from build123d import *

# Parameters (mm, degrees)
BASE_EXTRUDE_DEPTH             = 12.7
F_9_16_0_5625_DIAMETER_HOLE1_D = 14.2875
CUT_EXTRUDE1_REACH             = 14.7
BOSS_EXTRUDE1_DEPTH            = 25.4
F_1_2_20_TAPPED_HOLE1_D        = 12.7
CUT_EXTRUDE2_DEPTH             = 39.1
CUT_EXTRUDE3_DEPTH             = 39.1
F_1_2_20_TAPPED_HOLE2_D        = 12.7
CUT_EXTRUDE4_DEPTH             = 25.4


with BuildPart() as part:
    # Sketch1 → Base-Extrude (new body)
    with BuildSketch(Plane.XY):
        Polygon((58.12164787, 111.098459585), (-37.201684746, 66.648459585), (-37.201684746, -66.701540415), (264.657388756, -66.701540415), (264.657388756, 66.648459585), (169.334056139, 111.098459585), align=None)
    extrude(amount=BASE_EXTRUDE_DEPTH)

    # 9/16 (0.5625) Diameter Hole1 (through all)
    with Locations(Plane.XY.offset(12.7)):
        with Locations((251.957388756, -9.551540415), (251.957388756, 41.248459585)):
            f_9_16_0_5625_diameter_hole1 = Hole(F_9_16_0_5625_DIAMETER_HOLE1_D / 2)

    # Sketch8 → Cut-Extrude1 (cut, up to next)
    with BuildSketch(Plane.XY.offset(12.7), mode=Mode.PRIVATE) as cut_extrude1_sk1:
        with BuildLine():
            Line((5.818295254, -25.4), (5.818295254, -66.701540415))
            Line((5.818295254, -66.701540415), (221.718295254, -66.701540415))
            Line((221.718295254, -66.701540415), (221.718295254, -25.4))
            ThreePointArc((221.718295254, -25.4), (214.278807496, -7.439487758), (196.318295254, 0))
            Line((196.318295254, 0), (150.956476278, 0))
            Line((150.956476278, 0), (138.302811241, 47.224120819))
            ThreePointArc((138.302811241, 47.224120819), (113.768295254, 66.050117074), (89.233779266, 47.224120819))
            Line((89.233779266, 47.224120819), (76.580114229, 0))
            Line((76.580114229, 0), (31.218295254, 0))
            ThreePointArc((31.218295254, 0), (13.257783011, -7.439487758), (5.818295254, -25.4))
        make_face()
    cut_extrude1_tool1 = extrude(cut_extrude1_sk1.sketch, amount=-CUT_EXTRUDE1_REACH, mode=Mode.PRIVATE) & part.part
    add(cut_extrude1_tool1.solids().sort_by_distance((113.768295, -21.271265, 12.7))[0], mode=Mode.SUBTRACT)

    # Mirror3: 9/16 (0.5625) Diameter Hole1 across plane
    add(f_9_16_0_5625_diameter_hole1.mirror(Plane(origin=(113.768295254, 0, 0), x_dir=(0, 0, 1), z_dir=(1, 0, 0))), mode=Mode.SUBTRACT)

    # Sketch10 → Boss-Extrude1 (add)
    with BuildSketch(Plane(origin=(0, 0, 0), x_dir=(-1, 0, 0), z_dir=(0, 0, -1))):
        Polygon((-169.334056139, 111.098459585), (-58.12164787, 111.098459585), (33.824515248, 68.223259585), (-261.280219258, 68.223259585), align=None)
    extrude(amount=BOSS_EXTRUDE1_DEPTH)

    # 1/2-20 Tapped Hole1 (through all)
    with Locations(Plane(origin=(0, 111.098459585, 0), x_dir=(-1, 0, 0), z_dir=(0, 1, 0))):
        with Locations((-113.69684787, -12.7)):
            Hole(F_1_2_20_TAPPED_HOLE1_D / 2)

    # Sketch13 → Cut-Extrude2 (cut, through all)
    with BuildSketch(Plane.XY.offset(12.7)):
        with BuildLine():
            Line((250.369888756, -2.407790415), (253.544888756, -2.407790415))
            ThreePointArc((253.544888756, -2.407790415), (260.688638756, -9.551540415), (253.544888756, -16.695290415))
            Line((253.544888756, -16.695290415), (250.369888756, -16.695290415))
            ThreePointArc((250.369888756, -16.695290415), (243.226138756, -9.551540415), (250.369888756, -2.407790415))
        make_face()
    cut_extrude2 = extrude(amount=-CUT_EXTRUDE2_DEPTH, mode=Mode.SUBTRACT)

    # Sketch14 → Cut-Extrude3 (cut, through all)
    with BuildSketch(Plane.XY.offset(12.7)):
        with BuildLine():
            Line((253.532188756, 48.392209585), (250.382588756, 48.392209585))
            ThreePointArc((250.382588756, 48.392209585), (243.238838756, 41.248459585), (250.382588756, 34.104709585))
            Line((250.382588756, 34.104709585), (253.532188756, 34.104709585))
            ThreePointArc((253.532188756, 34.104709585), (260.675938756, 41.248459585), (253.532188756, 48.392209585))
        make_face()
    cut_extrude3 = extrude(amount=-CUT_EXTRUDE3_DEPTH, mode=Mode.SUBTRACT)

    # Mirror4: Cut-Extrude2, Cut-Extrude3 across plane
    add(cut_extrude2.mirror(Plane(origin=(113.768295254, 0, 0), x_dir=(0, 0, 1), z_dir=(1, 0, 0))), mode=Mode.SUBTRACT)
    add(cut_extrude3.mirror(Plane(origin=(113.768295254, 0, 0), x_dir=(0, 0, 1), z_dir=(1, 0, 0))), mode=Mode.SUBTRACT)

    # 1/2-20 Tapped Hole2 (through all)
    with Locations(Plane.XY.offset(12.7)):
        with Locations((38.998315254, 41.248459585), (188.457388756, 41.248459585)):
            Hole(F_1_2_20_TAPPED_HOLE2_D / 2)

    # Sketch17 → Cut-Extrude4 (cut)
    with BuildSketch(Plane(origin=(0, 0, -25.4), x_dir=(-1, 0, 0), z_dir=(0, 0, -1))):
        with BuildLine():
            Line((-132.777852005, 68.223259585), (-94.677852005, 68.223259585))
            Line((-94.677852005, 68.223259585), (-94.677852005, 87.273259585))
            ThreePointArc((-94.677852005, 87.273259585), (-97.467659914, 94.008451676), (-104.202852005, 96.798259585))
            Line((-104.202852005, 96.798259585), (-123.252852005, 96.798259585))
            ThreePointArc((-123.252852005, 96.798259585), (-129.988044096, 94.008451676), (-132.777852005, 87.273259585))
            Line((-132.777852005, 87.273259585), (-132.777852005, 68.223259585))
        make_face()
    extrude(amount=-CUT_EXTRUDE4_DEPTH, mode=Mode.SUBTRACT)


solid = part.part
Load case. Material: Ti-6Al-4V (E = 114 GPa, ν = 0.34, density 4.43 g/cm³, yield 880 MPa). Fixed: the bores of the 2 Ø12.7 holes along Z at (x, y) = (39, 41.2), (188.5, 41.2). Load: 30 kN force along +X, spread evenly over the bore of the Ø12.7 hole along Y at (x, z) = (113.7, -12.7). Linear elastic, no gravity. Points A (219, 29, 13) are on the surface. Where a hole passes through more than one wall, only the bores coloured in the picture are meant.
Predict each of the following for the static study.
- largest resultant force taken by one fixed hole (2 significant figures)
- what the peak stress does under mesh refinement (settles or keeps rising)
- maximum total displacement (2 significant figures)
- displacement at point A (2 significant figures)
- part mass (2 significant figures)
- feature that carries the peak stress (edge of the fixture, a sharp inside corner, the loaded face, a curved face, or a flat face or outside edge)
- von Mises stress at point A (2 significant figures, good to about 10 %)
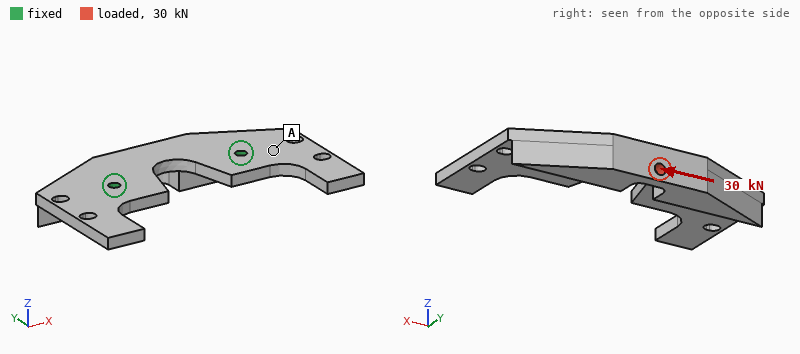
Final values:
19 kN
keeps rising
58 µm
15 µm
2.6 kg
edge of the fixture
14 MPa
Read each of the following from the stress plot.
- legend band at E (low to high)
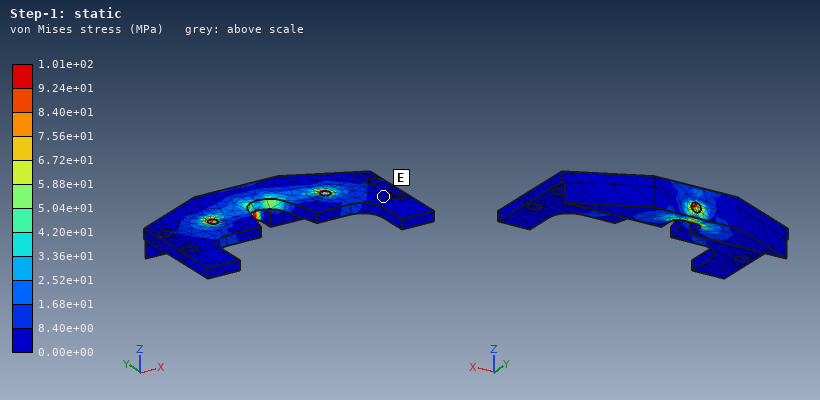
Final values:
0.00e+00 to 8.40e+00 MPa
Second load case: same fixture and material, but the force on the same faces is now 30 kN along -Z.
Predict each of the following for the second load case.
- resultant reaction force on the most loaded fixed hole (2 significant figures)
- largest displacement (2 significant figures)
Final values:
15 kN
1.1 mm
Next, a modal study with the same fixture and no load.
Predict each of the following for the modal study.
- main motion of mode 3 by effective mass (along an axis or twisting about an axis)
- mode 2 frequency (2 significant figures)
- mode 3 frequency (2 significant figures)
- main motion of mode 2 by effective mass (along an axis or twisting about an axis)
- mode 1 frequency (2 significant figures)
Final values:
along Z
830 Hz
1200 Hz
twisting about Y
790 Hz
